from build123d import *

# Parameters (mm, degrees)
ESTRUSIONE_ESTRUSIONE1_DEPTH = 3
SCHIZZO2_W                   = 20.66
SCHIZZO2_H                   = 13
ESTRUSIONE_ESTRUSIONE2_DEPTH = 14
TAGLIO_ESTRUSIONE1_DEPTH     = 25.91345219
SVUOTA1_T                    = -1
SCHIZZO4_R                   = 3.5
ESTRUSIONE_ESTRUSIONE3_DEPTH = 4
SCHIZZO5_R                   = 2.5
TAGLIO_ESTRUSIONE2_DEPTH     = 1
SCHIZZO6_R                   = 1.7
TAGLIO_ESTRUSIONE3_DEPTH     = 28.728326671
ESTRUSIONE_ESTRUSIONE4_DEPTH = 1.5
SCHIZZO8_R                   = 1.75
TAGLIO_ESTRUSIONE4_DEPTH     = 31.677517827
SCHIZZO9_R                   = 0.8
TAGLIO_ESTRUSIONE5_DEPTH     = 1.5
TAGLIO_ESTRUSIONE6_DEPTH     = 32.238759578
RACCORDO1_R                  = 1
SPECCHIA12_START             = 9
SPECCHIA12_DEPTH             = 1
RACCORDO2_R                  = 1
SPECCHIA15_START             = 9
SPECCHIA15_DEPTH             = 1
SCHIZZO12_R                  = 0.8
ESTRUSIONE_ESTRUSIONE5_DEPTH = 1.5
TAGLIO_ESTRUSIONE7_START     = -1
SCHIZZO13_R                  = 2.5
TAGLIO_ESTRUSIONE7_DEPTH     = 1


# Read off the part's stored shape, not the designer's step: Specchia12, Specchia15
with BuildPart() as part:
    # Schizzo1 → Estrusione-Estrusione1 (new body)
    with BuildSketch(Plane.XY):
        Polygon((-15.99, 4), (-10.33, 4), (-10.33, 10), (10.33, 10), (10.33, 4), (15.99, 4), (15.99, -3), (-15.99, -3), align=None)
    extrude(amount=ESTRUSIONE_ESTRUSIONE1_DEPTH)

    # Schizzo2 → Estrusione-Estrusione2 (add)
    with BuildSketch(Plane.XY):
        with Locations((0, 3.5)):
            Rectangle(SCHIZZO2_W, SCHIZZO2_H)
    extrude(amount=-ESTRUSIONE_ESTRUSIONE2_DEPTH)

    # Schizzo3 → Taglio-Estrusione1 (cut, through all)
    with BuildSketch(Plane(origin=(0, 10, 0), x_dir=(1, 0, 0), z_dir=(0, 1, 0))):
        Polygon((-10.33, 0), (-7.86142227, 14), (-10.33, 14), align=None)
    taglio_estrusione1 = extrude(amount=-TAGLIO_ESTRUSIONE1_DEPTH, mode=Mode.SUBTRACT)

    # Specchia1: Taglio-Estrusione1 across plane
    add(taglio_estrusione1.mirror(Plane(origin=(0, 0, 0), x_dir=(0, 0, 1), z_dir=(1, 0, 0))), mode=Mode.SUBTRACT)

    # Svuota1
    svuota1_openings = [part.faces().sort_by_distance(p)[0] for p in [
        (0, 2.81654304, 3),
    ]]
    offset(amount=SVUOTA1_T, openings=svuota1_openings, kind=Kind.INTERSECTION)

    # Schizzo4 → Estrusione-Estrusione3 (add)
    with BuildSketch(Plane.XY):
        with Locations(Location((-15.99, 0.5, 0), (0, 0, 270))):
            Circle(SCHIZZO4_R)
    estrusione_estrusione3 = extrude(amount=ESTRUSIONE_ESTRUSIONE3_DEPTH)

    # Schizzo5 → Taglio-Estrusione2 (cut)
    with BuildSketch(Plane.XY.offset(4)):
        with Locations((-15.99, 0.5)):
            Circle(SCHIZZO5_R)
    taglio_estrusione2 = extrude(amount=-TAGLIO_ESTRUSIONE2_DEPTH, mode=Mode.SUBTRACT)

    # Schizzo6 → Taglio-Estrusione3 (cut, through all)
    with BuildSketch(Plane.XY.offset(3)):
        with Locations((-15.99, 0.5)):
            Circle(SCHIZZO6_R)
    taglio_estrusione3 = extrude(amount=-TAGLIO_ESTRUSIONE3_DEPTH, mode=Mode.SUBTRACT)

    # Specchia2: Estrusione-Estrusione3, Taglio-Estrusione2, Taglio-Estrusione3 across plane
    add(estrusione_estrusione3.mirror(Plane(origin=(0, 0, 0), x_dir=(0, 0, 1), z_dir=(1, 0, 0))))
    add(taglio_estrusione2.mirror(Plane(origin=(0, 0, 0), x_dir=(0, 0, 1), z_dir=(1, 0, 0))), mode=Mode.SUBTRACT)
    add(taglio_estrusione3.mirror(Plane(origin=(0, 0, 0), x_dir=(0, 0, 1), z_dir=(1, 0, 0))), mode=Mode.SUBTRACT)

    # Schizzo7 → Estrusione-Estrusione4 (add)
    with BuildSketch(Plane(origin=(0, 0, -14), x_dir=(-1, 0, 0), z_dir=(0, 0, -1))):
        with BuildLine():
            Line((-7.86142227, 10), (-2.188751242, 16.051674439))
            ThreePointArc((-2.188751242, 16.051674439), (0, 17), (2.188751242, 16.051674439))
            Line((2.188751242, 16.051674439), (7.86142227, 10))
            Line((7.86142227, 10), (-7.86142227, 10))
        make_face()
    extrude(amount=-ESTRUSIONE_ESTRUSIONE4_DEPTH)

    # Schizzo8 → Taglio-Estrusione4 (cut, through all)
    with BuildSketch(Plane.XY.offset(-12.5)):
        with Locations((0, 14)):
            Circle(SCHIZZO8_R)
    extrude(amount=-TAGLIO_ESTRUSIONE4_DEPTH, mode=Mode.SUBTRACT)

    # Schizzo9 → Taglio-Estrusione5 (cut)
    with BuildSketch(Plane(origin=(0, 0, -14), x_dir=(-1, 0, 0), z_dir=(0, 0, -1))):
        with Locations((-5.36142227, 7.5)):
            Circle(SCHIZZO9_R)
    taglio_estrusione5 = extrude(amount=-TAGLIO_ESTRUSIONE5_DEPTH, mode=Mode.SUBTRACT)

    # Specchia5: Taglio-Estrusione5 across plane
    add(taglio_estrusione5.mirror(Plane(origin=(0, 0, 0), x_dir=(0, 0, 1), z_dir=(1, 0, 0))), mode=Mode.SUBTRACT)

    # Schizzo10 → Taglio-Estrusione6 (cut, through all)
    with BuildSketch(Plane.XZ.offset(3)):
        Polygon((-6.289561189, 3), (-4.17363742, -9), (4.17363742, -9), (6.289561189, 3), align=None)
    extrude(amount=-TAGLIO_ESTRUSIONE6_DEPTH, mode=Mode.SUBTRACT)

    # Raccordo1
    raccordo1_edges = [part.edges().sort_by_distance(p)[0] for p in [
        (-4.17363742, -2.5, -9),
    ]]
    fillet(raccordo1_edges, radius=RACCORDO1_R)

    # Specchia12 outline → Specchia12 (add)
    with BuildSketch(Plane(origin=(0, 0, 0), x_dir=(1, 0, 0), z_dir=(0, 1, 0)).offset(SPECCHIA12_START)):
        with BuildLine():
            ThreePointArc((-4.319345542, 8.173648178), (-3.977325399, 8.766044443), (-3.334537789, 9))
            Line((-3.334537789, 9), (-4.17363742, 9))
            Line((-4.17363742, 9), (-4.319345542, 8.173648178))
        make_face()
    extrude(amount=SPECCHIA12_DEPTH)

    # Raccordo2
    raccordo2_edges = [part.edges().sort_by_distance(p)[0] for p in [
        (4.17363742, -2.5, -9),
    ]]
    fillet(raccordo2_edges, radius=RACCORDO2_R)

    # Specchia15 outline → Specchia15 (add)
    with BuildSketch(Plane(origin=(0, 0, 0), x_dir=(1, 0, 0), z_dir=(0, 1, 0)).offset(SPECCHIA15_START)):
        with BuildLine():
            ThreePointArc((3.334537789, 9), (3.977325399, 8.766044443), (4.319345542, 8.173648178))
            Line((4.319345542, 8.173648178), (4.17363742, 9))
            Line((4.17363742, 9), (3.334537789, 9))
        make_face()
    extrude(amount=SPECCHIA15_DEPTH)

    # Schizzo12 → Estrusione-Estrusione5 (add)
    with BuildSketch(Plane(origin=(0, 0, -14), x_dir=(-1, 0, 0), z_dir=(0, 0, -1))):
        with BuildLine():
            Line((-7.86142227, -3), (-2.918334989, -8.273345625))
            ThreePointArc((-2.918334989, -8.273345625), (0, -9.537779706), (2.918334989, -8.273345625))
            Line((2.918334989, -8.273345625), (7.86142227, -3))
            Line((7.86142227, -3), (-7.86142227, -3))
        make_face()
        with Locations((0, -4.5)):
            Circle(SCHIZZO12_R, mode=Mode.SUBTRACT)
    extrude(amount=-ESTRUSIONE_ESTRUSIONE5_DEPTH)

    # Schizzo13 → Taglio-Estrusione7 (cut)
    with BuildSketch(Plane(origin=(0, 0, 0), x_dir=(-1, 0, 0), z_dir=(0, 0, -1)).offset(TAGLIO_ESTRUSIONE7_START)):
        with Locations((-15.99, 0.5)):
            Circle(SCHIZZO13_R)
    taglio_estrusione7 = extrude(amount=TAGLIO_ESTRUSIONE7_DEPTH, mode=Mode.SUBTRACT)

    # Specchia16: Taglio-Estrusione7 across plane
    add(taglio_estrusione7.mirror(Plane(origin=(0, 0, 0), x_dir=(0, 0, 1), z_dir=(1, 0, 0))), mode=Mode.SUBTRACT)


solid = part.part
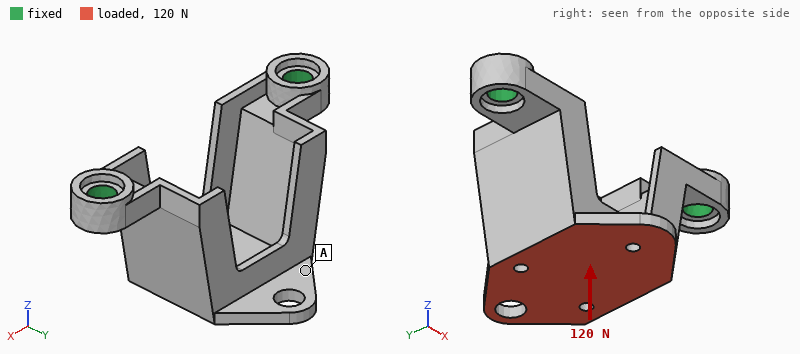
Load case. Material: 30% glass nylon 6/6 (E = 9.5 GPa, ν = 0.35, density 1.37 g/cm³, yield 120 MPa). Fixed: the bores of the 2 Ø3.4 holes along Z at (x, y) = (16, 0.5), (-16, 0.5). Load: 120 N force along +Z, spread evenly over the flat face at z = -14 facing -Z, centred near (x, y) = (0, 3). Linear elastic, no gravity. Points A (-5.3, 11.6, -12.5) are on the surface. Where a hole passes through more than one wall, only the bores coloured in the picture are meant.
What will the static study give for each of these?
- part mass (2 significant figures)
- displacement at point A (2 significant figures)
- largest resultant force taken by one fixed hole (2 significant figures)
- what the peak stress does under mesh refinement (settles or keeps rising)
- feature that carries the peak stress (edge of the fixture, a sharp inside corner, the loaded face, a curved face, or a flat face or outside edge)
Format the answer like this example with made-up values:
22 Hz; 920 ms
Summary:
1.8 g; 0.27 mm; 66 N; keeps rising; a sharp inside corner
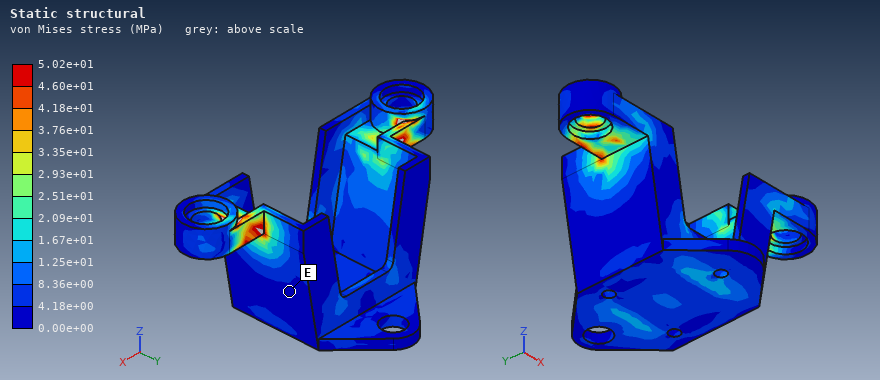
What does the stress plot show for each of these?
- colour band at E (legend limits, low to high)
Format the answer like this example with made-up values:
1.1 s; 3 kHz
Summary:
0.00e+00 to 4.18e+00 MPa
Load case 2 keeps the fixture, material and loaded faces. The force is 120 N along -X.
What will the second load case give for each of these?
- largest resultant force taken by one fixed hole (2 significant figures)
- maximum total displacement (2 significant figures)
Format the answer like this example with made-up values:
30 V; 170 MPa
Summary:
96 N; 0.21 mm
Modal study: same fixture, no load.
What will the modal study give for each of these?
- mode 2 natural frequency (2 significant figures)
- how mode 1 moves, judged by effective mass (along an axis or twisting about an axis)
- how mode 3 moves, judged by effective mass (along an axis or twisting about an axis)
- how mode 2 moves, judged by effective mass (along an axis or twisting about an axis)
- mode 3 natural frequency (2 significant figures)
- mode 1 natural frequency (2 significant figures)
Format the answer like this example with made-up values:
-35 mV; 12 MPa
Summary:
3400 Hz; along Y; along X; along X; 5800 Hz; 1700 Hz
